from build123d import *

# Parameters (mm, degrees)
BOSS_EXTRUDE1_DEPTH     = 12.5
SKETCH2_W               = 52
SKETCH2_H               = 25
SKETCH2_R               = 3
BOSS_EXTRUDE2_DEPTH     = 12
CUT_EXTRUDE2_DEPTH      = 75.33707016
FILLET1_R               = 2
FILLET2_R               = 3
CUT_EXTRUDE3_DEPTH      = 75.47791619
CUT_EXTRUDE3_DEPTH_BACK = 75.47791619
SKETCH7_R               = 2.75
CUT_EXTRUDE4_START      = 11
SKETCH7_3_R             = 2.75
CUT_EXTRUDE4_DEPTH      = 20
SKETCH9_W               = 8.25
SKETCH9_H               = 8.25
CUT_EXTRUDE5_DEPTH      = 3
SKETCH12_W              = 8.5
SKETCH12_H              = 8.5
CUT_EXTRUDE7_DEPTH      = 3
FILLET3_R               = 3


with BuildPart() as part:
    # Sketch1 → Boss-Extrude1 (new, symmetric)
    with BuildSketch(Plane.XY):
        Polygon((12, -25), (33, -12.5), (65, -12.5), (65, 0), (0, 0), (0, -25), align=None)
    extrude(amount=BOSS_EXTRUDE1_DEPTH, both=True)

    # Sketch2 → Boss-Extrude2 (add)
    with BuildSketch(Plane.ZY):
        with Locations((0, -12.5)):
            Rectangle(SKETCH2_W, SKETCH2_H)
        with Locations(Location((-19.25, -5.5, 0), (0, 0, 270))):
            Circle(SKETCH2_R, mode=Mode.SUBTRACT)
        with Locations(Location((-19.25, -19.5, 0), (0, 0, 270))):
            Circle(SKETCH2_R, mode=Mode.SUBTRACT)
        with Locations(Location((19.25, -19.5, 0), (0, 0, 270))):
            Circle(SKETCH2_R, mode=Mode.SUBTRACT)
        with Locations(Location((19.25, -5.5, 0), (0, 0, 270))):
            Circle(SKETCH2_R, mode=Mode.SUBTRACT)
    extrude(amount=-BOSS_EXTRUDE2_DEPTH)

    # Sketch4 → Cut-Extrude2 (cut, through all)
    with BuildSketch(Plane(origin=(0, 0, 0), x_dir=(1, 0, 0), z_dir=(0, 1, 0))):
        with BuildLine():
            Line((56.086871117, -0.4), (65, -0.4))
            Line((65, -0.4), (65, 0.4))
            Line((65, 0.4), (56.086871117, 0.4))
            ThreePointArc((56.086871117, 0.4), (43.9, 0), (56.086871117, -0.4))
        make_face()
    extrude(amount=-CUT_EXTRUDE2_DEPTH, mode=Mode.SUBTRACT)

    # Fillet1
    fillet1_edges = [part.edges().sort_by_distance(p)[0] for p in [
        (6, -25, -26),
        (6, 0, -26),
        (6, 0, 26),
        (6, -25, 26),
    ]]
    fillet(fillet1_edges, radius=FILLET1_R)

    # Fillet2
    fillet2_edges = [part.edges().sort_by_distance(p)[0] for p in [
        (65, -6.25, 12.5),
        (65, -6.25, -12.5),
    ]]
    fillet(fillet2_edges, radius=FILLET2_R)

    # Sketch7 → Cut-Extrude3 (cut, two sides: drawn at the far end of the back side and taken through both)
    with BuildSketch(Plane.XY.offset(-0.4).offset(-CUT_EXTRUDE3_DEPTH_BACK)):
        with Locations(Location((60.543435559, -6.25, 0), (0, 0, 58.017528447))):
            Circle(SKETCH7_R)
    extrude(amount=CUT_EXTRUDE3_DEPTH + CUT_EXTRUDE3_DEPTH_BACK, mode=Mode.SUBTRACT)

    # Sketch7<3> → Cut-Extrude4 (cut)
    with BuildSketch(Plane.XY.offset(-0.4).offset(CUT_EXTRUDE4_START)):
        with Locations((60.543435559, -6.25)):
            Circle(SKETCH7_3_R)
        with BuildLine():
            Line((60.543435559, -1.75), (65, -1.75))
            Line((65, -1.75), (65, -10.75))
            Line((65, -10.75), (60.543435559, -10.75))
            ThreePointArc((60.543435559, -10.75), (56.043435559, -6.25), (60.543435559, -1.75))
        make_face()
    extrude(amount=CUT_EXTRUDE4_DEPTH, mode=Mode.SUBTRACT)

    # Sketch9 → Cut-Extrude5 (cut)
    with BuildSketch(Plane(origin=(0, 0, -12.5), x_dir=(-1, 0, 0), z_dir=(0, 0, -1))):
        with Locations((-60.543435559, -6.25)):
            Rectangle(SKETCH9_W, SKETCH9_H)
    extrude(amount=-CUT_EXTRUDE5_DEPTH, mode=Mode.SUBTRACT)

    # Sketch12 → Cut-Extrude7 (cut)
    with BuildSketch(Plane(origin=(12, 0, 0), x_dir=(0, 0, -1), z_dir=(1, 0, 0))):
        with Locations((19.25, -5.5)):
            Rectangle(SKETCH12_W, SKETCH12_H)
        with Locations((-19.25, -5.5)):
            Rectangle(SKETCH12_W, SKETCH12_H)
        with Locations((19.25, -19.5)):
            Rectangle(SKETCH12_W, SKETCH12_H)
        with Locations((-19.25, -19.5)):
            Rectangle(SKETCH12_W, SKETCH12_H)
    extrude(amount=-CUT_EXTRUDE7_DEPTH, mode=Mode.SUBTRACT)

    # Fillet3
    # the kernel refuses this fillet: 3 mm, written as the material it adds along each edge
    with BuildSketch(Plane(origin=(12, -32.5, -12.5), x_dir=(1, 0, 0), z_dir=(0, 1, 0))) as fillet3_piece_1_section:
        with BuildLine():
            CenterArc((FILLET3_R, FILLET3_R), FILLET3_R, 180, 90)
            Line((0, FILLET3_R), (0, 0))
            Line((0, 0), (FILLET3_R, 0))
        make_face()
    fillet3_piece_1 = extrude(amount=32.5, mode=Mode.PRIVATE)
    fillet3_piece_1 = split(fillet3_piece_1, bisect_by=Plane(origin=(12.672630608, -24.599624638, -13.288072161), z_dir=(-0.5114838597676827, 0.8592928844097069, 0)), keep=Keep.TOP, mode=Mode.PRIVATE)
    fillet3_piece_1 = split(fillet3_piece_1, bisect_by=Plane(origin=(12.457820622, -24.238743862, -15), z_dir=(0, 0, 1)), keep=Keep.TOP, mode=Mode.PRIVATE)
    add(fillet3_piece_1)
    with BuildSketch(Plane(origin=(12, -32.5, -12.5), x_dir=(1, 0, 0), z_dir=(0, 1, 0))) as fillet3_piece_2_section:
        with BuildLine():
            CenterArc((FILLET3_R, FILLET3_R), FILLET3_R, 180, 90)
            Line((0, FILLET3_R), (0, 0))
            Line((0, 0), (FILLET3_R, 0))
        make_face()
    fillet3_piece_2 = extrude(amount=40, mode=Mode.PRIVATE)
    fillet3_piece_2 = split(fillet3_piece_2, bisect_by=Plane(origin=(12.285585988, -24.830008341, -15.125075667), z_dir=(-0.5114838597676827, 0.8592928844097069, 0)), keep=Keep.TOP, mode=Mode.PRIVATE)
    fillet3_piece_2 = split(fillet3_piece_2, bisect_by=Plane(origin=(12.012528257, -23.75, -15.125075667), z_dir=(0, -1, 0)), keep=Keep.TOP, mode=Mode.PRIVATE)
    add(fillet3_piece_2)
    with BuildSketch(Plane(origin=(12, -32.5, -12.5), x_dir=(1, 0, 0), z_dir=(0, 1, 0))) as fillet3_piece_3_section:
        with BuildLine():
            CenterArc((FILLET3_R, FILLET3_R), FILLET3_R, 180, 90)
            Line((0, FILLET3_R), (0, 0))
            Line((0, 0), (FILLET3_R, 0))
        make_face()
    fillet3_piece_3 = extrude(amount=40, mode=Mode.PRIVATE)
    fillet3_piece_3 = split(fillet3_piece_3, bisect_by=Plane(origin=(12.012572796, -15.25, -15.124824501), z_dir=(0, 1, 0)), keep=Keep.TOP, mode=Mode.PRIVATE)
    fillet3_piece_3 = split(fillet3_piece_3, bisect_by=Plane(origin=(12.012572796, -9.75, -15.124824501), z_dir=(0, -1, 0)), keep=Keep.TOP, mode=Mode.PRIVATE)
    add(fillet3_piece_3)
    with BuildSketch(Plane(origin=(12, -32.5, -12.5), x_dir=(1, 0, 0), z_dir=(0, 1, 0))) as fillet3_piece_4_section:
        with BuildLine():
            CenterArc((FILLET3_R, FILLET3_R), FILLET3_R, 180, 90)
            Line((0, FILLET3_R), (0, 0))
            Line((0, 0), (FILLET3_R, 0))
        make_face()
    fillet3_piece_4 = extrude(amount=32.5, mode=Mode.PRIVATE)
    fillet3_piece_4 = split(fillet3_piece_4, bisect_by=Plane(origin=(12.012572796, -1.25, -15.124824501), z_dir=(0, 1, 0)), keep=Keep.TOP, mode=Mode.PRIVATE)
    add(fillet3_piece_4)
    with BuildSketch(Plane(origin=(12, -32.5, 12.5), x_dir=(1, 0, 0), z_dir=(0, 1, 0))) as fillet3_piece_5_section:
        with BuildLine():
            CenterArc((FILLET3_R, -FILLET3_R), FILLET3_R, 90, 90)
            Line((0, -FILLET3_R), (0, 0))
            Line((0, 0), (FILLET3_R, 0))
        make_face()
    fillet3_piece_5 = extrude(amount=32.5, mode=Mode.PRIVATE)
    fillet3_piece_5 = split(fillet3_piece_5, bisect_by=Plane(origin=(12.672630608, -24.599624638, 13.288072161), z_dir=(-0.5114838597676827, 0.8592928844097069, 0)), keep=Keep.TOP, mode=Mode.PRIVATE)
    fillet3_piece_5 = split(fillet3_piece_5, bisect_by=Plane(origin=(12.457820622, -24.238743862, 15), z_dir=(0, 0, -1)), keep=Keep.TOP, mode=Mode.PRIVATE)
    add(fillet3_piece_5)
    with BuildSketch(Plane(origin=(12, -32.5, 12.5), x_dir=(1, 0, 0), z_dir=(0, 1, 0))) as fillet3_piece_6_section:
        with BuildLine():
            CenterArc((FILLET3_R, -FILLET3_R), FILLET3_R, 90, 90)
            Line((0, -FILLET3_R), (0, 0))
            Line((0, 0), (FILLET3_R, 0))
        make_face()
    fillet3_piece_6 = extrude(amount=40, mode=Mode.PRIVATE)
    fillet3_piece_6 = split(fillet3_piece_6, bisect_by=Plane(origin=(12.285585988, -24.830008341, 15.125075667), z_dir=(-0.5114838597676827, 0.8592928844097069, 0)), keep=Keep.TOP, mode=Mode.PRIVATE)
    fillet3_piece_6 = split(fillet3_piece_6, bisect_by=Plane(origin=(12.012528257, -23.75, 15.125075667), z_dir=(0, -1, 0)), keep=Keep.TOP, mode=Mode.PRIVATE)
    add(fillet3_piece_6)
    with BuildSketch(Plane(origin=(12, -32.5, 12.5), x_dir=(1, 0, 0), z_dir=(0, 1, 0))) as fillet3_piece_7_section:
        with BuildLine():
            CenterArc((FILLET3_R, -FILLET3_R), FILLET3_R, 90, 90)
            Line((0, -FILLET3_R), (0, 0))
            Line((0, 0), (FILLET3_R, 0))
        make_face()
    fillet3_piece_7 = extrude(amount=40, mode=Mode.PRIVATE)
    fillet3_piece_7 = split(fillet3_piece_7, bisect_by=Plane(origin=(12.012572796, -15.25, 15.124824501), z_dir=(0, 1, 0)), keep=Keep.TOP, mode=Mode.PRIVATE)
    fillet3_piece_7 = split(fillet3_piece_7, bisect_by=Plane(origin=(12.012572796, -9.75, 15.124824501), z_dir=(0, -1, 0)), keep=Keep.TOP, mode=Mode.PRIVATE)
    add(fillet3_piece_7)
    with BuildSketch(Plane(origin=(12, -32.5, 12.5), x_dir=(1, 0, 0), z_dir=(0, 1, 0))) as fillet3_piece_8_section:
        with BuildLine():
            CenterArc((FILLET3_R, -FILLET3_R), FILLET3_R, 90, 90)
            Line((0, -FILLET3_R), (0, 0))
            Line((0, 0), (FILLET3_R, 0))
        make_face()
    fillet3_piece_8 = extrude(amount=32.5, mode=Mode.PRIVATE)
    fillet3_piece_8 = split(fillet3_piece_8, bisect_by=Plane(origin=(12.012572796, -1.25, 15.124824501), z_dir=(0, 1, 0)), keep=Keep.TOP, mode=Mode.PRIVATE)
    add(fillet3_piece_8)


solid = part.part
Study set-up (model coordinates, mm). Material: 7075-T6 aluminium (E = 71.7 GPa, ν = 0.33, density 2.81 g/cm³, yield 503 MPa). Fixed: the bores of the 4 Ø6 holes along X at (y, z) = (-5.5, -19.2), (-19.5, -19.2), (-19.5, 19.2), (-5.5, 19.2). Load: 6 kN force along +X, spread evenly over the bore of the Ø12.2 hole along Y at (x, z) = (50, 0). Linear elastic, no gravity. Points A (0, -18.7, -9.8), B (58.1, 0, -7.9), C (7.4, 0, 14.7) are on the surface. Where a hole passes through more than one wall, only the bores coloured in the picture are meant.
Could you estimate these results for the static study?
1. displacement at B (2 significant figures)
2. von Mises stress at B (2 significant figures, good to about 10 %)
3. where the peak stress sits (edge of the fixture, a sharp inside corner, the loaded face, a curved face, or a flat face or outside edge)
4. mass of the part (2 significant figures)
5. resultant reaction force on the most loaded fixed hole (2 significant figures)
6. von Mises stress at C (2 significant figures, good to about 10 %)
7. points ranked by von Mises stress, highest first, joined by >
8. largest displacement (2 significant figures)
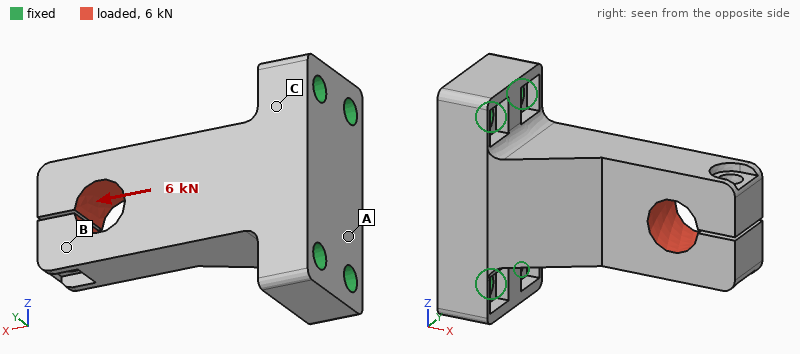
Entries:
0.059 mm
21 MPa
the loaded face
88 g
2.7 kN
54 MPa
C > B > A
0.10 mm
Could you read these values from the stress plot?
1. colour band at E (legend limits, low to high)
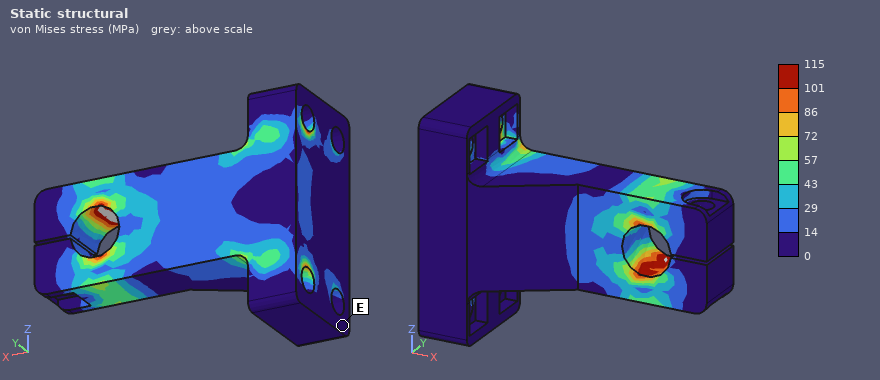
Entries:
0 to 14 MPa
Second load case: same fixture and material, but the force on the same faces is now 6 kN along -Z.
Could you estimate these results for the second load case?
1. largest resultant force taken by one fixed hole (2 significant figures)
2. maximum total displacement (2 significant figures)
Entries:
4.9 kN
0.27 mm
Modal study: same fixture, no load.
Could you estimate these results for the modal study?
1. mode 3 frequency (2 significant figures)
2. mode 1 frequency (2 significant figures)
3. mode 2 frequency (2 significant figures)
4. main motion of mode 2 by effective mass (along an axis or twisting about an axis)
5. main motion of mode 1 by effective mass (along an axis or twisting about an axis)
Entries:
8700 Hz
4600 Hz
6200 Hz
along Z
along Y
